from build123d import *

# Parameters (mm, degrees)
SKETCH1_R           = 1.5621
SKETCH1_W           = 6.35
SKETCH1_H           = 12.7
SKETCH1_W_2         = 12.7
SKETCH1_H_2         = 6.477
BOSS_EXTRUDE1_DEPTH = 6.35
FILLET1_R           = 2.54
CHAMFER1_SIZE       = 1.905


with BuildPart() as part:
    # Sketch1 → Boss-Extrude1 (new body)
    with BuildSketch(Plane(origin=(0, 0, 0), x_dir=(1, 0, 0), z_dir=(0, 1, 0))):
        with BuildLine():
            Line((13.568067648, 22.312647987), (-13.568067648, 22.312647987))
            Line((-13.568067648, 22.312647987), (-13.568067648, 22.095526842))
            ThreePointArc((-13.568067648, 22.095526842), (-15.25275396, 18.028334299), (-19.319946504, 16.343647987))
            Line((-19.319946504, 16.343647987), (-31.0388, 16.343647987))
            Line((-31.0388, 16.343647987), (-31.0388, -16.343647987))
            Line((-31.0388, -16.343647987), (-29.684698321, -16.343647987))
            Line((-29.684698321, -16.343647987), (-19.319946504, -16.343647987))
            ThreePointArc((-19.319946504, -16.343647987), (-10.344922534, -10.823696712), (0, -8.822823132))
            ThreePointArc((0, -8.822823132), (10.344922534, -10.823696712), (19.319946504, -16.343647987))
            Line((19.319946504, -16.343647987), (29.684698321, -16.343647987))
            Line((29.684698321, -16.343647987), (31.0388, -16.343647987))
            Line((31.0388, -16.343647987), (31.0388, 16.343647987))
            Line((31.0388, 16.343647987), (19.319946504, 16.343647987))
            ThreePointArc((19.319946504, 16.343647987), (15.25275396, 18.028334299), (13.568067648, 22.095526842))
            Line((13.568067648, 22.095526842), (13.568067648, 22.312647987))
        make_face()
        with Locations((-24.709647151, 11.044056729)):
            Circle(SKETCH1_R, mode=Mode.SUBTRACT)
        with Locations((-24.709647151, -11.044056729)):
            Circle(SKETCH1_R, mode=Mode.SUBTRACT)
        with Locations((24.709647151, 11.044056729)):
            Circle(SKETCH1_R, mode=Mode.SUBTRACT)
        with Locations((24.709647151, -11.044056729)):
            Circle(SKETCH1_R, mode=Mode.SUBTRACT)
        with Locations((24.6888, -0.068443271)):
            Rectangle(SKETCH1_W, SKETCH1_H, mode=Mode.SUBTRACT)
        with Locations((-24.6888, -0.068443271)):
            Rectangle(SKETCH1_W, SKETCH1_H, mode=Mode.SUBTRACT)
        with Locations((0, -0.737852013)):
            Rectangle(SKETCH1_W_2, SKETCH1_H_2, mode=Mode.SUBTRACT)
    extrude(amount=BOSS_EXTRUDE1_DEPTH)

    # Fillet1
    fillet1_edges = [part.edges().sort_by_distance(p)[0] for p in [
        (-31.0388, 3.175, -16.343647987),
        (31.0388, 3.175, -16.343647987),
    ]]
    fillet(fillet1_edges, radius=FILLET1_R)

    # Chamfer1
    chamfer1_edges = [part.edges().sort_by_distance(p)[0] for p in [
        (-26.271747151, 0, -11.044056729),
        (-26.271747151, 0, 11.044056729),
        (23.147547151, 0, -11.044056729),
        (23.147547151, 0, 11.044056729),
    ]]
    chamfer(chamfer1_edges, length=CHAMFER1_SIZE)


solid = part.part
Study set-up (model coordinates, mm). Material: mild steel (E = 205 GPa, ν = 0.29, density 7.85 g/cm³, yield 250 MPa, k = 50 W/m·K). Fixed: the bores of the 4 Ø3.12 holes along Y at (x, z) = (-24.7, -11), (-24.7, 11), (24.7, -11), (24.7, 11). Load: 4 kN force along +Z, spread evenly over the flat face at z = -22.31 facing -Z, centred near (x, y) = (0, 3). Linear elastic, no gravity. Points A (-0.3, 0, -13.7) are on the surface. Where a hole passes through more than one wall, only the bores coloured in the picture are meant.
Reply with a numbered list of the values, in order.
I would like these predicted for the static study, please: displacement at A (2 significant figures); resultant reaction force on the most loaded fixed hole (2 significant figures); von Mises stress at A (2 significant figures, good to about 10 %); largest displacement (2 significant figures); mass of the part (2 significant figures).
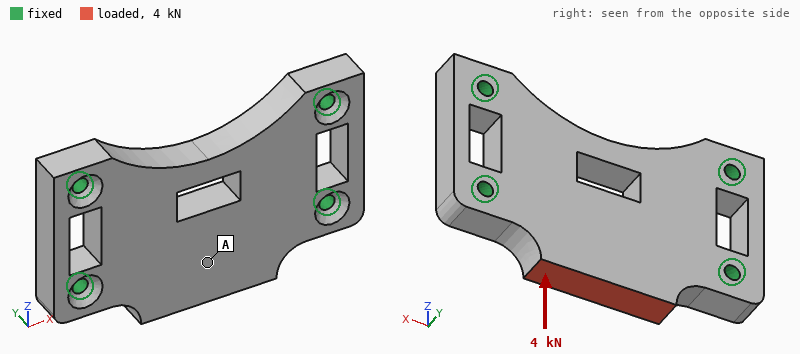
1. 5.2 µm
2. 1.2 kN
3. 15 MPa
4. 5.9 µm
5. 85 g
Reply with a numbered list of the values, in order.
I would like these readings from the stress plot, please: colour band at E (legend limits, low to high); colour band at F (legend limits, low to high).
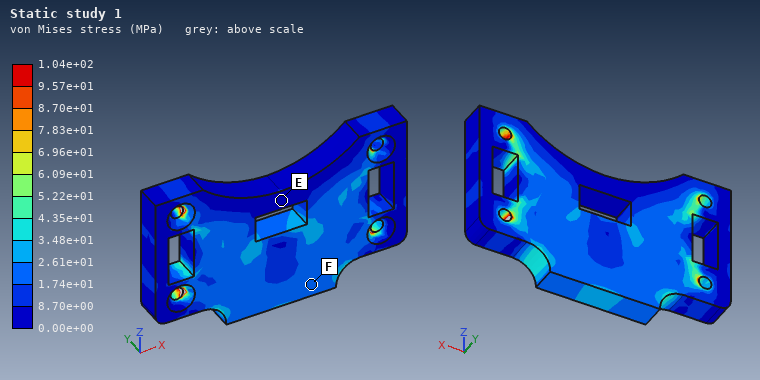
1. 0.00e+00 to 8.70e+00 MPa
2. 1.74e+01 to 2.61e+01 MPa
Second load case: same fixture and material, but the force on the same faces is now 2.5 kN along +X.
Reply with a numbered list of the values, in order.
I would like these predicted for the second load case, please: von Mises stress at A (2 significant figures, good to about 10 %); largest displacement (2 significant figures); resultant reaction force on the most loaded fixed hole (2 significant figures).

1. 12 MPa
2. 3.9 µm
3. 1.2 kN
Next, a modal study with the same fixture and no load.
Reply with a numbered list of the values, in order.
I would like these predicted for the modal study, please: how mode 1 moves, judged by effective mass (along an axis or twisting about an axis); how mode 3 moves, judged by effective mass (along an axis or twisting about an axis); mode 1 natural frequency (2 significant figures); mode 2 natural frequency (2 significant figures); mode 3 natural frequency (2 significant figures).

1. along Y
2. along Z
3. 9300 Hz
4. 14 kHz
5. 23 kHz
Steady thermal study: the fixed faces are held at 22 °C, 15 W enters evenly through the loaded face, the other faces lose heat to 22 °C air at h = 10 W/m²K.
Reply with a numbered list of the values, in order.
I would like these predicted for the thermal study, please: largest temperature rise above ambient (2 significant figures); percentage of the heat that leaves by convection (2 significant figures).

1. 38 K
2. 3.3 %
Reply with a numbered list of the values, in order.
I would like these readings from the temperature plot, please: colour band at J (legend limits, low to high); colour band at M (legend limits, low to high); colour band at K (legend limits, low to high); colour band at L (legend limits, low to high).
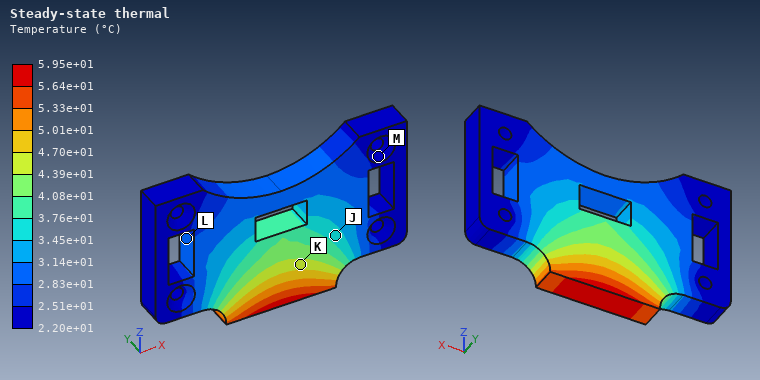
1. 3.45e+01 to 3.76e+01 °C
2. 2.20e+01 to 2.51e+01 °C
3. 4.39e+01 to 4.70e+01 °C
4. 2.83e+01 to 3.14e+01 °C
